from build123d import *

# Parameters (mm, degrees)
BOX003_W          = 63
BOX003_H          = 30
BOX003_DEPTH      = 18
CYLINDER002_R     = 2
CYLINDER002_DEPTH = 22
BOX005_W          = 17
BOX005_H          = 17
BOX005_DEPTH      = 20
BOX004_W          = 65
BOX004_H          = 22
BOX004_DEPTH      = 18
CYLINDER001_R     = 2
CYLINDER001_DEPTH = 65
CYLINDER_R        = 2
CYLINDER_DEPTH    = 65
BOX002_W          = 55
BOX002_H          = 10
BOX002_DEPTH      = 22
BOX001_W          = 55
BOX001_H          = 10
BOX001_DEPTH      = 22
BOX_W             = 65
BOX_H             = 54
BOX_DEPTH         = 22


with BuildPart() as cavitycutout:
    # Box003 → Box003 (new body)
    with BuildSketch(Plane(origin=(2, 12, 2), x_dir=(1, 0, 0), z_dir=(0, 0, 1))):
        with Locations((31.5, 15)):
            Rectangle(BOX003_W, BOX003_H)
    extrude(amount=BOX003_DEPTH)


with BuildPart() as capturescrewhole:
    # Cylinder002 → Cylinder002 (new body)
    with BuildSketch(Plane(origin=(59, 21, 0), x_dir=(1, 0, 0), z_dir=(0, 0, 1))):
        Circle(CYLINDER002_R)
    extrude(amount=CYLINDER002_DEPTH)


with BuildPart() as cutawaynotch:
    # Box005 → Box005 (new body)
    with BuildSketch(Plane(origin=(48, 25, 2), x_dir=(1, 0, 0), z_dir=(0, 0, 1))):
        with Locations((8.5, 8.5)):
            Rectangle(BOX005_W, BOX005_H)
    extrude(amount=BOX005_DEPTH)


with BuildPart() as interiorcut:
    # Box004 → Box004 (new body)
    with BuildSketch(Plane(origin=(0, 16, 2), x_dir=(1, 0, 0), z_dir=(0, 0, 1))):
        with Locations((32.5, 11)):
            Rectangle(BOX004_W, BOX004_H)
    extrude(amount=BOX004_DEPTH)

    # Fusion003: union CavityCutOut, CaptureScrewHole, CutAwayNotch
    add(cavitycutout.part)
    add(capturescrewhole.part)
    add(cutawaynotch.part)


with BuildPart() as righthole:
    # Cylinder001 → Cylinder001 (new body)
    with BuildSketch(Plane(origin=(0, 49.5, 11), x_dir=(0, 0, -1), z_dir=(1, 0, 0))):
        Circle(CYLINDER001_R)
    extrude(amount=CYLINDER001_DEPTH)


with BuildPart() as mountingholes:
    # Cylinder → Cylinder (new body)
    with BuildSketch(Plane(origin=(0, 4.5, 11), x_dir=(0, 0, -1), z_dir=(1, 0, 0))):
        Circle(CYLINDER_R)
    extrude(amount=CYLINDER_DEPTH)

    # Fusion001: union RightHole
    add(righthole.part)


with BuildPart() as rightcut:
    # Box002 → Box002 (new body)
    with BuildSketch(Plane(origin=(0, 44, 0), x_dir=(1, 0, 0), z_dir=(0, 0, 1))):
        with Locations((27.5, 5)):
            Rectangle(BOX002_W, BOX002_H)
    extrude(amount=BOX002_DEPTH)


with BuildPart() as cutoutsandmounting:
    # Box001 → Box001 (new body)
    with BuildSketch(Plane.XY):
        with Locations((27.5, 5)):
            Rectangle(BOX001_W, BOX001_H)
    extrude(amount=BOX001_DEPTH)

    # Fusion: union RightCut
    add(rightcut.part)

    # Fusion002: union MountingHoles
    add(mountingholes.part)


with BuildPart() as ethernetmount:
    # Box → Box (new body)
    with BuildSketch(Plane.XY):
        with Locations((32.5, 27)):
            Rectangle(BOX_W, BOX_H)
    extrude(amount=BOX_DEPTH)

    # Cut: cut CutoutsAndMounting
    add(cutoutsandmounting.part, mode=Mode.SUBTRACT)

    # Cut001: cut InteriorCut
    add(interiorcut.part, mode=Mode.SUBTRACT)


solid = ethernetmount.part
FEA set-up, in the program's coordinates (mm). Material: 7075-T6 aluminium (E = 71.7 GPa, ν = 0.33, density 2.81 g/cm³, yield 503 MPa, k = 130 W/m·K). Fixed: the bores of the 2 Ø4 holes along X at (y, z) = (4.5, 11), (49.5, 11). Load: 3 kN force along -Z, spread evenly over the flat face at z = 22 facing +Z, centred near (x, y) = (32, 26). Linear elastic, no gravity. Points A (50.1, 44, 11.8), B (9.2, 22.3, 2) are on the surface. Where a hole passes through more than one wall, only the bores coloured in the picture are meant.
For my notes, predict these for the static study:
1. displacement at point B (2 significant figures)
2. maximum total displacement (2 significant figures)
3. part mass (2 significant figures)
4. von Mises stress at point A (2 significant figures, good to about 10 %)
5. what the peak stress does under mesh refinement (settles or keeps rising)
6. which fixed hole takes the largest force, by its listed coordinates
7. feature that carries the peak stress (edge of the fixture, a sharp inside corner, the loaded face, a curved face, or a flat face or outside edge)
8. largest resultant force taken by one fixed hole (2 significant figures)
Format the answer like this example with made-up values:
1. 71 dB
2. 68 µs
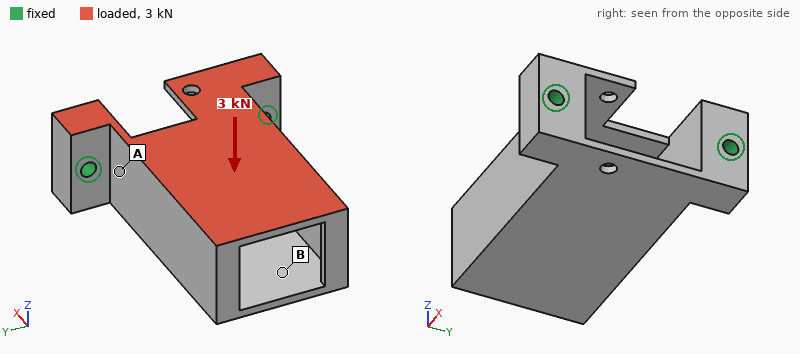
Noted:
1. 0.29 mm
2. 0.42 mm
3. 49 g
4. 73 MPa
5. keeps rising
6. (4.5, 11)
7. edge of the fixture
8. 1.7 kN
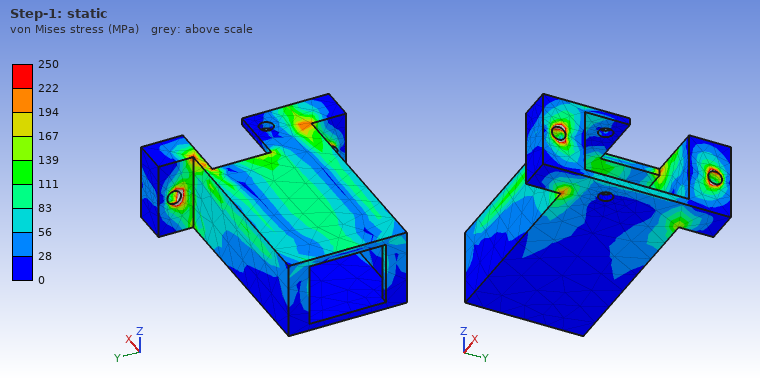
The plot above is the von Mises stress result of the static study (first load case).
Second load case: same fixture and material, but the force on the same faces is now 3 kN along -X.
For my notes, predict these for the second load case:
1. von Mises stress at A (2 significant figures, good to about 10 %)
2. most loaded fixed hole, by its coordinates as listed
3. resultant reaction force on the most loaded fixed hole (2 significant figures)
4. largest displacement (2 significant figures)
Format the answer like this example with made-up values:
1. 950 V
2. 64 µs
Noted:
1. 36 MPa
2. (4.5, 11)
3. 1.7 kN
4. 0.15 mm
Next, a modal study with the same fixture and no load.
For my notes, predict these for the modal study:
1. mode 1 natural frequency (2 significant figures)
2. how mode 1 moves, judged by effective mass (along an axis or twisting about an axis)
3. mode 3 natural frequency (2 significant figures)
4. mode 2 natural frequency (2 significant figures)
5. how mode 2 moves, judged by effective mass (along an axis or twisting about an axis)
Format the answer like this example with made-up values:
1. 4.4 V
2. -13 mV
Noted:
1. 2700 Hz
2. along Z
3. 5600 Hz
4. 5300 Hz
5. along Y
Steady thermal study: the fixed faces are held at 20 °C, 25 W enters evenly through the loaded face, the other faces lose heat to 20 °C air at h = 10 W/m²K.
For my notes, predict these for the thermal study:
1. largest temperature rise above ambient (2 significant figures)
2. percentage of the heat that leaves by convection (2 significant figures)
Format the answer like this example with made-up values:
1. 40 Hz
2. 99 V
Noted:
1. 37 K
2. 9.5 %
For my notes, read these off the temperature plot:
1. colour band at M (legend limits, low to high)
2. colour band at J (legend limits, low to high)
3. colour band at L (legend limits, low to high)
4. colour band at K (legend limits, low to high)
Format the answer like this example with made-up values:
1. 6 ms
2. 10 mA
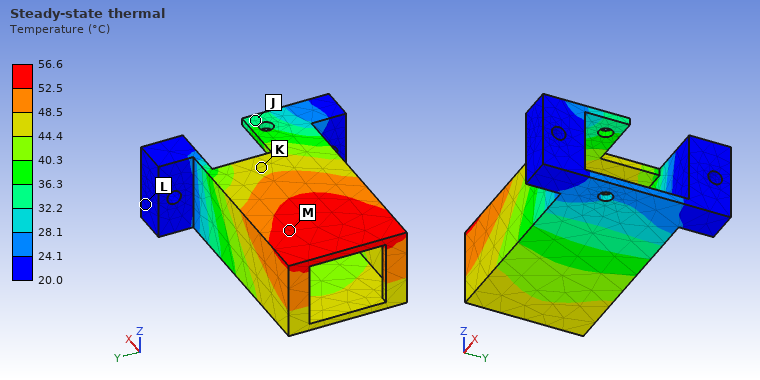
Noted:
1. 52.5 to 56.6 °C
2. 32.2 to 36.3 °C
3. 20.0 to 24.1 °C
4. 44.4 to 48.5 °C
